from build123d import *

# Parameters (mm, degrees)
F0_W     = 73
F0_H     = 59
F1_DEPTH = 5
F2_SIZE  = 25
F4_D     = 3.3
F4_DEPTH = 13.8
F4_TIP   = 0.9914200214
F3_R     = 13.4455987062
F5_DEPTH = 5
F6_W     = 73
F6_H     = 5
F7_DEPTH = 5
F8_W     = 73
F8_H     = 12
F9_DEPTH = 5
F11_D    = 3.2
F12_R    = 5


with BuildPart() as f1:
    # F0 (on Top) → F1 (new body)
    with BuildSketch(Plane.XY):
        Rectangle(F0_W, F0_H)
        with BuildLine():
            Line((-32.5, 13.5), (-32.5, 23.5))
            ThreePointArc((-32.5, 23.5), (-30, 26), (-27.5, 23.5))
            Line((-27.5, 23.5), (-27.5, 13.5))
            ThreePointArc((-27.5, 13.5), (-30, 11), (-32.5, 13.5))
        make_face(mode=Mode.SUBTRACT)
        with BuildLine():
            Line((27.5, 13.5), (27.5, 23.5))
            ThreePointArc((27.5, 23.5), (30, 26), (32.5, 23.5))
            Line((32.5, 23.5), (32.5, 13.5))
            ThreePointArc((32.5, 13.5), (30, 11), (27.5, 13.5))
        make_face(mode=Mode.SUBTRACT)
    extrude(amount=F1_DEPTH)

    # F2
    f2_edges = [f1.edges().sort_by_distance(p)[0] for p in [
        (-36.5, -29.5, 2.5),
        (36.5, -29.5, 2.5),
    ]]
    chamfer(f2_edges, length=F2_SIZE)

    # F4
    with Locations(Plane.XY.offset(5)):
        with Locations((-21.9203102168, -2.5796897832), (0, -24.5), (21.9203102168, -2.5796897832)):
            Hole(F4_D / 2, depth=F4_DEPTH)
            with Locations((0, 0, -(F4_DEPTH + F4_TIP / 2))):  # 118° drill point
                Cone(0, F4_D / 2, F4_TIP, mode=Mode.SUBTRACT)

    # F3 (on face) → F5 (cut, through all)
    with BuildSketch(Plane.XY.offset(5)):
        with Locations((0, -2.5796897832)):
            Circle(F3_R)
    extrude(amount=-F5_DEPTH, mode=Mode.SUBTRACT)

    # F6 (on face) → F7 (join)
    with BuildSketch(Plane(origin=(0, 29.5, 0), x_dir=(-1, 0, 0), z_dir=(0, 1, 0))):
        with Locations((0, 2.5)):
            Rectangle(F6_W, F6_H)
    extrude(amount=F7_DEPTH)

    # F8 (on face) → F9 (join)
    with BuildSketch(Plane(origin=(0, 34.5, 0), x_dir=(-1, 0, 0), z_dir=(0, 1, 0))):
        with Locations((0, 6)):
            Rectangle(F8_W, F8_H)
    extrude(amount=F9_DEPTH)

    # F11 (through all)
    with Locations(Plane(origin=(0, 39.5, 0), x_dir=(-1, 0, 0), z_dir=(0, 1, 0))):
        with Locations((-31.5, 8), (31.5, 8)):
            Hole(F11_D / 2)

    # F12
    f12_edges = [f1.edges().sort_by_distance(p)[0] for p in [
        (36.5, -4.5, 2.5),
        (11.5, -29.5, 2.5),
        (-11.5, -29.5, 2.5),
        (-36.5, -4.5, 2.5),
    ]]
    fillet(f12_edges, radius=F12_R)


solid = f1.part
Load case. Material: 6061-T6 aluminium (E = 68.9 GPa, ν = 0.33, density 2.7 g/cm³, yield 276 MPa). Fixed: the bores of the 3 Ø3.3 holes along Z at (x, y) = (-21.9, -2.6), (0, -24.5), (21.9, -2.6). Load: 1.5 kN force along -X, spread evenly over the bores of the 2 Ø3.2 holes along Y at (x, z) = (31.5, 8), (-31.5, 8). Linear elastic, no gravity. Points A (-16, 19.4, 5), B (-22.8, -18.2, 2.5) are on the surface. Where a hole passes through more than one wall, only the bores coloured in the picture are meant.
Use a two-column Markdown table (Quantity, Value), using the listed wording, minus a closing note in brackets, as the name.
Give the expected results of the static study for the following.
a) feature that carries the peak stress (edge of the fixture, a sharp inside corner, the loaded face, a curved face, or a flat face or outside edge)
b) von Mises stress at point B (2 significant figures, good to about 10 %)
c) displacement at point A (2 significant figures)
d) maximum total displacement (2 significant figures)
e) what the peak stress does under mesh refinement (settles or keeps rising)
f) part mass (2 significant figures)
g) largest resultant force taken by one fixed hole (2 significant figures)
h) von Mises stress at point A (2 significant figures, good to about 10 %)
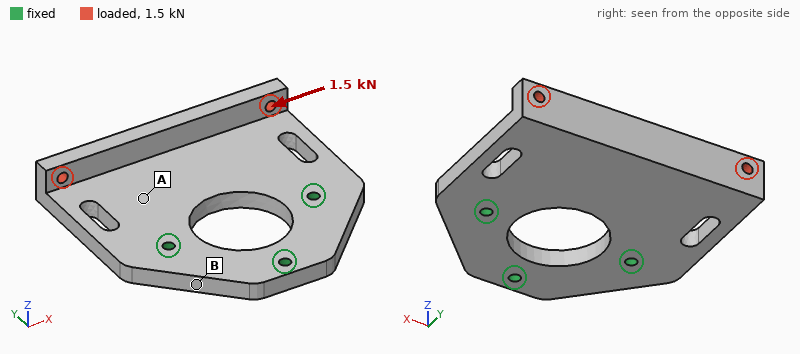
| Quantity | Value |
|---|---|
| feature that carries the peak stress | edge of the fixture |
| von Mises stress at point B | 10 MPa |
| displacement at point A | 0.025 mm |
| maximum total displacement | 0.11 mm |
| what the peak stress does under mesh refinement | keeps rising |
| part mass | 56 g |
| largest resultant force taken by one fixed hole | 1.4 kN |
| von Mises stress at point A | 25 MPa |
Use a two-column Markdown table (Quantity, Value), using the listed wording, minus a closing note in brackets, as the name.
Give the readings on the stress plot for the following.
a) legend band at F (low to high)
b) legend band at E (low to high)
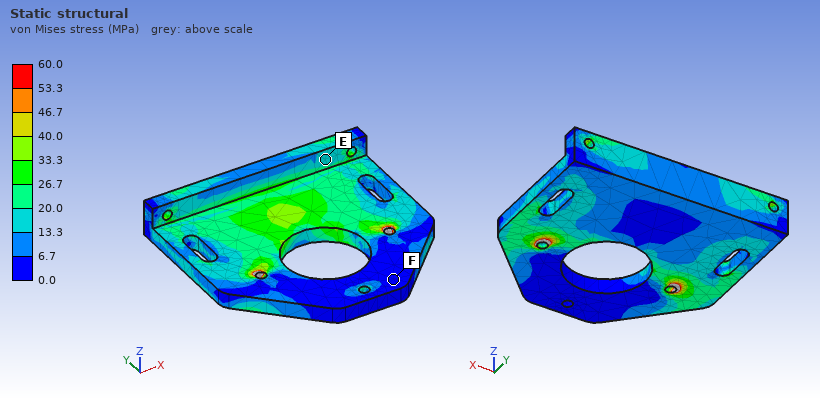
| Quantity | Value |
|---|---|
| legend band at F | 0.0 to 6.7 MPa |
| legend band at E | 13.3 to 20.0 MPa |
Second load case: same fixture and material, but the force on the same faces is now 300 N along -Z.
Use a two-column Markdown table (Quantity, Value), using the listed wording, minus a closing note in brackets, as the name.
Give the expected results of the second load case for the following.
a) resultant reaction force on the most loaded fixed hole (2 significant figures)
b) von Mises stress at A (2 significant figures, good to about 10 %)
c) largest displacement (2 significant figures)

| Quantity | Value |
|---|---|
| resultant reaction force on the most loaded fixed hole | 180 N |
| von Mises stress at A | 19 MPa |
| largest displacement | 0.23 mm |
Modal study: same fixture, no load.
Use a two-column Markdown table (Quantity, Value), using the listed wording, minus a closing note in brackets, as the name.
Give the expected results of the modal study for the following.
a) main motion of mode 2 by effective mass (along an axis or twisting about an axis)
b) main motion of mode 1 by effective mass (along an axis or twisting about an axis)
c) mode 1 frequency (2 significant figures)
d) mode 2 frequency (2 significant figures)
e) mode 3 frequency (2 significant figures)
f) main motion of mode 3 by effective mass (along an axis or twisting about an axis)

| Quantity | Value |
|---|---|
| main motion of mode 2 by effective mass | twisting about Y |
| main motion of mode 1 by effective mass | along Z |
| mode 1 frequency | 1400 Hz |
| mode 2 frequency | 2900 Hz |
| mode 3 frequency | 8700 Hz |
| main motion of mode 3 by effective mass | along X |
